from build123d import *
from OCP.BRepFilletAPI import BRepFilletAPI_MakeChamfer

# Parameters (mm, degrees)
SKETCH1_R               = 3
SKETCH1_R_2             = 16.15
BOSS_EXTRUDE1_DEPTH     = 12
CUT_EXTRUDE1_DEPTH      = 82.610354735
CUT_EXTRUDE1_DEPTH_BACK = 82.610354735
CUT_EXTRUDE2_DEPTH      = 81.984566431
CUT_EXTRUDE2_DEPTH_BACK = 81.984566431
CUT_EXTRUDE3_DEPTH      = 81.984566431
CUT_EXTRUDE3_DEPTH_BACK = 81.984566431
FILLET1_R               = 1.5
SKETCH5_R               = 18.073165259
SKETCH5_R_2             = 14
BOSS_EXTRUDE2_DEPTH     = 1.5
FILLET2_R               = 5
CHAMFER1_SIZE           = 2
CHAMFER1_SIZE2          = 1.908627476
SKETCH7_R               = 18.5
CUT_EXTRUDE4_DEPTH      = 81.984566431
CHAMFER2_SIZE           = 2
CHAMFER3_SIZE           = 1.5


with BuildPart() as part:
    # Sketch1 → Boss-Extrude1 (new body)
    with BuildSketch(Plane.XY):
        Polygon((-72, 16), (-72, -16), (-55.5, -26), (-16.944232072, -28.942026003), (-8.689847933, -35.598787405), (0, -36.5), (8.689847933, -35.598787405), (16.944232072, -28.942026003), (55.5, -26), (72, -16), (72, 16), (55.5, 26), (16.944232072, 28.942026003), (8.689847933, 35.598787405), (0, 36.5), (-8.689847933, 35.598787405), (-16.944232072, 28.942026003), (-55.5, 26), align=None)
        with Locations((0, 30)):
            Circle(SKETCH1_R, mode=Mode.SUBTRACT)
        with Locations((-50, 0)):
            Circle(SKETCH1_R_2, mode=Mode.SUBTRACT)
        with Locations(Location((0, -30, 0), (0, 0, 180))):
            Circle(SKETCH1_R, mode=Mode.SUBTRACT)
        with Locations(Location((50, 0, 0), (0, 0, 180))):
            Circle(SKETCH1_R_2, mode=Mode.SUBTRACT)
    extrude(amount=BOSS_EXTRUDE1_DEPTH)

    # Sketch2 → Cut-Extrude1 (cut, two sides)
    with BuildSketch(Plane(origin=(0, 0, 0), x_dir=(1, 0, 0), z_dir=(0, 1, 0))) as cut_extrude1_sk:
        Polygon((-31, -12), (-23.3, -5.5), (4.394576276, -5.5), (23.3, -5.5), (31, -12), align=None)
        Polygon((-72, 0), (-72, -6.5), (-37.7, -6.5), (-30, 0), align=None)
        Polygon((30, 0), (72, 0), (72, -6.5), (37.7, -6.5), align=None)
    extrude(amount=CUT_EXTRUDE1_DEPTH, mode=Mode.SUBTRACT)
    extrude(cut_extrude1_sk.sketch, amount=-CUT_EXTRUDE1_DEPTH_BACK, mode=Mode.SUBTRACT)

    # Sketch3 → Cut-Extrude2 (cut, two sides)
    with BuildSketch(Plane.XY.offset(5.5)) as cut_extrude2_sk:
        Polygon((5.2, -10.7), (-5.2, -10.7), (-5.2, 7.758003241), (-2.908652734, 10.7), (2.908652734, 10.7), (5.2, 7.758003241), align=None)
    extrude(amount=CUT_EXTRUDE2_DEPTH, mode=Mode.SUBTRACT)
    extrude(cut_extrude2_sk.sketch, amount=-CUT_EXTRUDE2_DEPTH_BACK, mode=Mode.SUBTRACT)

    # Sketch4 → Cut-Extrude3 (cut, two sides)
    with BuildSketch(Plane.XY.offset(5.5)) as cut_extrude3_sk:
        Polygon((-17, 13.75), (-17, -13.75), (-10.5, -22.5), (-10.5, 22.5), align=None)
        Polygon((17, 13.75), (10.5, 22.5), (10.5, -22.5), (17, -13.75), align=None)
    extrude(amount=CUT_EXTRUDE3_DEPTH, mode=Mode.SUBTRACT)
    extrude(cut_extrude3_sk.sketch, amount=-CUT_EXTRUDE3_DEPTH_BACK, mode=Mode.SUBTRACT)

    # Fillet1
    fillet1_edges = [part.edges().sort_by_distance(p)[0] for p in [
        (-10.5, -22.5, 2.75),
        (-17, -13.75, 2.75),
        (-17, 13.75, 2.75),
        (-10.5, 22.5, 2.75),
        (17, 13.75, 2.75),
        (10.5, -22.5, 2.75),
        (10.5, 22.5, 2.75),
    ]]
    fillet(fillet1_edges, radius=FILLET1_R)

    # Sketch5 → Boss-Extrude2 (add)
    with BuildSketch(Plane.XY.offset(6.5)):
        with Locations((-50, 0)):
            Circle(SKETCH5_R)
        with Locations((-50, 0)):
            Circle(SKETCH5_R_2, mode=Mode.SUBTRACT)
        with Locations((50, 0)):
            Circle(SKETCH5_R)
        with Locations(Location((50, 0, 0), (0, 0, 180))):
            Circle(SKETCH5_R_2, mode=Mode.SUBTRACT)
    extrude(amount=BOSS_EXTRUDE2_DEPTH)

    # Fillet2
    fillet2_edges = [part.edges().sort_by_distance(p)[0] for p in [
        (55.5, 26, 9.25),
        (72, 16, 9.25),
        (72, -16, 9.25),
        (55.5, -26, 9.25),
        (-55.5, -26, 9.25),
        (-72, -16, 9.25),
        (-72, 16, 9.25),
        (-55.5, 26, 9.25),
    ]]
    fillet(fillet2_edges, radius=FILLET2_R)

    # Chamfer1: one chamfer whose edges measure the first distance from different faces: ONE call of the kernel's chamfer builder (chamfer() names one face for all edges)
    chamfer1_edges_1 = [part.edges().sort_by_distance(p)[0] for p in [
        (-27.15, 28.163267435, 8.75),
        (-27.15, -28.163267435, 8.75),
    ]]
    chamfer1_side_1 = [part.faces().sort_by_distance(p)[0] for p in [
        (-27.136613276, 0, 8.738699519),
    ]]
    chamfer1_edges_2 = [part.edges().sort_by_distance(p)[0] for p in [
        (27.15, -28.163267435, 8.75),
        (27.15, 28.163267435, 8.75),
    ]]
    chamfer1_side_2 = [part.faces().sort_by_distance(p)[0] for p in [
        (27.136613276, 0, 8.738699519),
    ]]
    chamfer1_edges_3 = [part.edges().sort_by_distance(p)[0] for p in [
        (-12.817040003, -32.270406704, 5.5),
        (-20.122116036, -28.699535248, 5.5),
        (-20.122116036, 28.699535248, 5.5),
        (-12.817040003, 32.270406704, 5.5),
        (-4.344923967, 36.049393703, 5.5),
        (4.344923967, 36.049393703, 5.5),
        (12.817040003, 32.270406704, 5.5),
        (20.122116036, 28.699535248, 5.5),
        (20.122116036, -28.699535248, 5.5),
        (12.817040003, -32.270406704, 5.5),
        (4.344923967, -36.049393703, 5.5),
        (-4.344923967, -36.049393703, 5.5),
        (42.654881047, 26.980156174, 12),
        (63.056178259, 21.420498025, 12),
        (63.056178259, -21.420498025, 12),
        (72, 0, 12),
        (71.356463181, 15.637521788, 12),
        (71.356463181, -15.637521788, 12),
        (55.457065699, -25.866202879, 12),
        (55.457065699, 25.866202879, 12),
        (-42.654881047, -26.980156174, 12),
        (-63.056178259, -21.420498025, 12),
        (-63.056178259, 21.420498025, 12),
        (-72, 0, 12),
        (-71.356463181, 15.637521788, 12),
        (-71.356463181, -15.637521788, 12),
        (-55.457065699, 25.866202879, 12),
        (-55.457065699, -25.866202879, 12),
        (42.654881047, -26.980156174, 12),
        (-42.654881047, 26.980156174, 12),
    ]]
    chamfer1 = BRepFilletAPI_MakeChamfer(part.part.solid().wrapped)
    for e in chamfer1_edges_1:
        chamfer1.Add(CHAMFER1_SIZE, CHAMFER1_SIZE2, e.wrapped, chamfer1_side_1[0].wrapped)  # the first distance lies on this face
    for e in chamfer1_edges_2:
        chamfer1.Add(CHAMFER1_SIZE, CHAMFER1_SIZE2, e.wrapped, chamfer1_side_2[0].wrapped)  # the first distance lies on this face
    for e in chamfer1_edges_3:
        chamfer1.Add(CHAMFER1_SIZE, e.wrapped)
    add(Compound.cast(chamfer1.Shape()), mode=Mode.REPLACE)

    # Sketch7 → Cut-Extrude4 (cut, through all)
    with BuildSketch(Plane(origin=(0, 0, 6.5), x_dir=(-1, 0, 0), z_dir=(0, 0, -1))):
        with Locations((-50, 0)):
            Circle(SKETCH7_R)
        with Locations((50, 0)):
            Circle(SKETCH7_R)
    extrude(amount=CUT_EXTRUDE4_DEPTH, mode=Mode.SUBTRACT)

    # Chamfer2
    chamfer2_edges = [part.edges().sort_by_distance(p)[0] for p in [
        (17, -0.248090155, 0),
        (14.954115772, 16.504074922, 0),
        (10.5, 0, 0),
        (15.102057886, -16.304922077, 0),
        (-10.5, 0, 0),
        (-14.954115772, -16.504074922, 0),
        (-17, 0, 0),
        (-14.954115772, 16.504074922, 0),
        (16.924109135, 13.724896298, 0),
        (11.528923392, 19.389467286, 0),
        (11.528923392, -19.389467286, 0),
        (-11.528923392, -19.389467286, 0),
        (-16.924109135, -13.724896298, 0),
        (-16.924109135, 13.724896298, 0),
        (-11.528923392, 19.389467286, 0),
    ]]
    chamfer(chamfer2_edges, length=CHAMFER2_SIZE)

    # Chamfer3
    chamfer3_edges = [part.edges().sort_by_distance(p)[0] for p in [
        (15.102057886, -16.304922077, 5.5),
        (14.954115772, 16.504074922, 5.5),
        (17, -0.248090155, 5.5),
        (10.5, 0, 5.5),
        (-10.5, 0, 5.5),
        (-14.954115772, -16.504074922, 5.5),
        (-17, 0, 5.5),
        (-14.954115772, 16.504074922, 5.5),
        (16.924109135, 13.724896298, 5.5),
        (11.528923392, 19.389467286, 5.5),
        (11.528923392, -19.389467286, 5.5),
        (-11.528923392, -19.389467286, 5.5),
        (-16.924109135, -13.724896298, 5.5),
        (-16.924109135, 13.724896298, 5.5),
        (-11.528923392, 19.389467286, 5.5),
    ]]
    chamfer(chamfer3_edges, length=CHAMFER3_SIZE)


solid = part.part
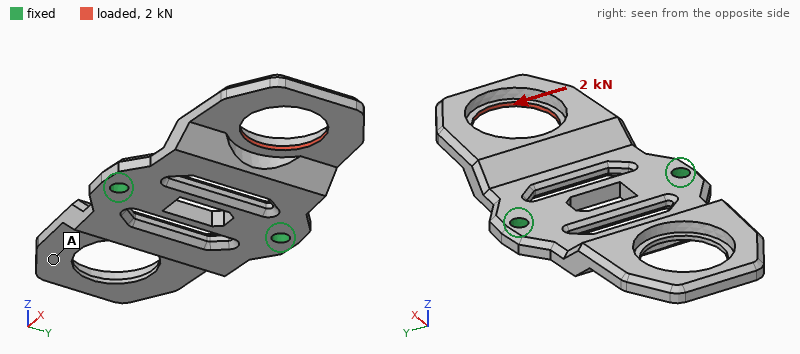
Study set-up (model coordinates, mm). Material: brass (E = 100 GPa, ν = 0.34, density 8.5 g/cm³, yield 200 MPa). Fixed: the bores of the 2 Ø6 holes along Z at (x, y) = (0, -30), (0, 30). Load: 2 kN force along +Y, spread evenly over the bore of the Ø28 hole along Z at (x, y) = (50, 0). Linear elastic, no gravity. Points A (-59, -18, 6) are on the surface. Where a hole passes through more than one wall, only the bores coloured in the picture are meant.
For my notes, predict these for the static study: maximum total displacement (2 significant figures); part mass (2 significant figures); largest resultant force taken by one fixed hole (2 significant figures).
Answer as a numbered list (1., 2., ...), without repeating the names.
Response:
1. 67 µm
2. 290 g
3. 1.8 kN
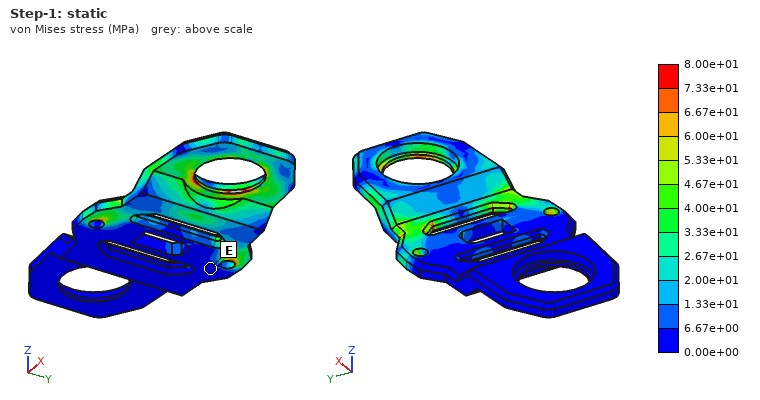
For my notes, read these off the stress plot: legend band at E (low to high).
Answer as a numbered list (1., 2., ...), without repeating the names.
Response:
1. 0.00e+00 to 6.67e+00 MPa
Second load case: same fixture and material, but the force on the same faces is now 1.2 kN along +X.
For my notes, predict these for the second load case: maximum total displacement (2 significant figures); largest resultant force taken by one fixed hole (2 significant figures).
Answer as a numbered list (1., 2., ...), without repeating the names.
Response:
1. 0.20 mm
2. 620 N
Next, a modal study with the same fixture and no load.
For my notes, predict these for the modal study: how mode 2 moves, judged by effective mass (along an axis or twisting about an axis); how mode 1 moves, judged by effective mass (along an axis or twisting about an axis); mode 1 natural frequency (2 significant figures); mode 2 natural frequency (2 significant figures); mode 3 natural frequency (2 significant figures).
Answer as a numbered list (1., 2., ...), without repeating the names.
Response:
1. along Z
2. twisting about Y
3. 570 Hz
4. 600 Hz
5. 2100 Hz
